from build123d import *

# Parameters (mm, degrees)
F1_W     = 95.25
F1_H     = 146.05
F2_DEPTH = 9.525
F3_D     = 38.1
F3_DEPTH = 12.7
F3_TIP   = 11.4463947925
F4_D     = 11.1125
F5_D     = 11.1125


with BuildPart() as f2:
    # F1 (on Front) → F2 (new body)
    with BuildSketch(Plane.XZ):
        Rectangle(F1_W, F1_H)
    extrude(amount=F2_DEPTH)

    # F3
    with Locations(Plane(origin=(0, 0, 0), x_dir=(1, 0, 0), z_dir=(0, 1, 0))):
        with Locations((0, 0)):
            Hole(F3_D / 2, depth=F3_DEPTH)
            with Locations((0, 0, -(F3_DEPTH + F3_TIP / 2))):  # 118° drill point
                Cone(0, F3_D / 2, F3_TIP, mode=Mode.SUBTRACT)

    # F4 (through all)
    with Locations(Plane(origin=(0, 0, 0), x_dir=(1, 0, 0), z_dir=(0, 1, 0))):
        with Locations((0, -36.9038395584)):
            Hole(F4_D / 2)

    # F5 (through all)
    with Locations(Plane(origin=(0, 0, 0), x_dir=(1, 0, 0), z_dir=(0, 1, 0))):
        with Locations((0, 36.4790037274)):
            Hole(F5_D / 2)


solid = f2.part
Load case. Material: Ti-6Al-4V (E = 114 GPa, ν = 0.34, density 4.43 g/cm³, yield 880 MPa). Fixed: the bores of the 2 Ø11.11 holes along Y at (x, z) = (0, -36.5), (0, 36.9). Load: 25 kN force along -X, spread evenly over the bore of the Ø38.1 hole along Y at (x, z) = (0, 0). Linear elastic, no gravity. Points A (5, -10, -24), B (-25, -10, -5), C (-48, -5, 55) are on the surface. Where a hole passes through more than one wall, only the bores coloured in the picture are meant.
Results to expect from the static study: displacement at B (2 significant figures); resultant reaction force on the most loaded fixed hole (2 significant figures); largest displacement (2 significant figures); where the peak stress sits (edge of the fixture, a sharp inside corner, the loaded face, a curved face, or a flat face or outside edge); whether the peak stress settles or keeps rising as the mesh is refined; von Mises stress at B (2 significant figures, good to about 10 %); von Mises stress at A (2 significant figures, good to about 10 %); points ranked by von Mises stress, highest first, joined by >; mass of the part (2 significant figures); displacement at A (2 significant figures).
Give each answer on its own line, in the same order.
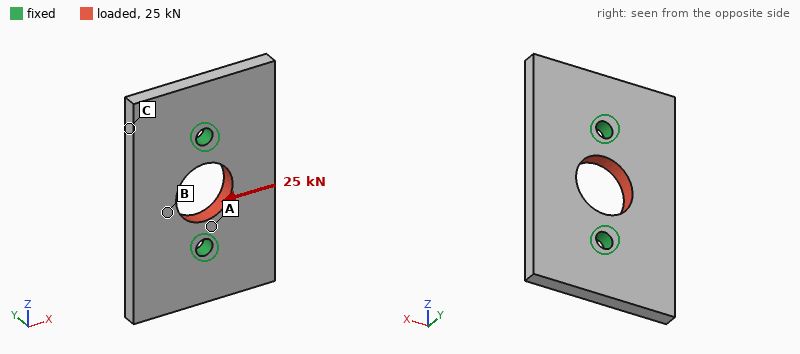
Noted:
13 µm
13 kN
15 µm
edge of the fixture
keeps rising
23 MPa
42 MPa
A > B > C
530 g
6.4 µm
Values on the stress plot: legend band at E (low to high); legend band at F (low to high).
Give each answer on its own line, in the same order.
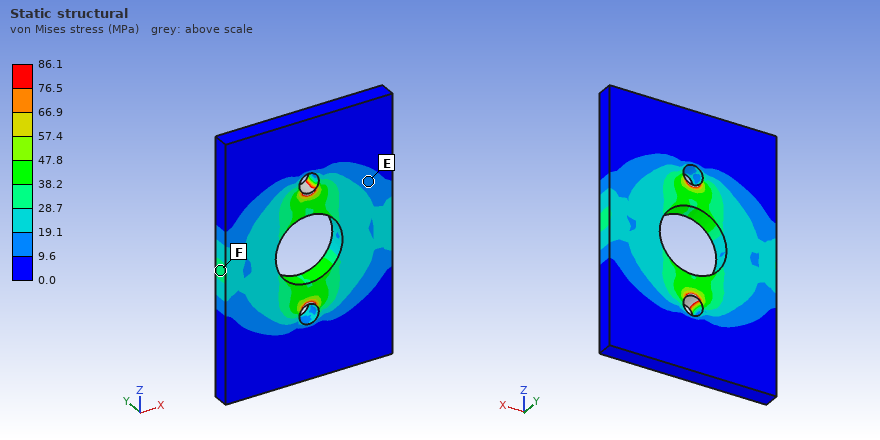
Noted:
9.6 to 19.1 MPa
28.7 to 38.2 MPa
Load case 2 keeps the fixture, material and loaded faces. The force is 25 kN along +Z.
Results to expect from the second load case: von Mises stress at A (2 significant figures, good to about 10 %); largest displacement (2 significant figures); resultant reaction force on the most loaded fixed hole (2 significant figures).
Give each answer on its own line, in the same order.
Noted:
40 MPa
11 µm
13 kN
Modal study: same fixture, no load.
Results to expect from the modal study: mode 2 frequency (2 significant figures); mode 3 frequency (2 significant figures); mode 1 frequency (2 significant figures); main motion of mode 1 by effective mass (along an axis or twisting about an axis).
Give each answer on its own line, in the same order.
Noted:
3200 Hz
3300 Hz
2700 Hz
twisting about Z
